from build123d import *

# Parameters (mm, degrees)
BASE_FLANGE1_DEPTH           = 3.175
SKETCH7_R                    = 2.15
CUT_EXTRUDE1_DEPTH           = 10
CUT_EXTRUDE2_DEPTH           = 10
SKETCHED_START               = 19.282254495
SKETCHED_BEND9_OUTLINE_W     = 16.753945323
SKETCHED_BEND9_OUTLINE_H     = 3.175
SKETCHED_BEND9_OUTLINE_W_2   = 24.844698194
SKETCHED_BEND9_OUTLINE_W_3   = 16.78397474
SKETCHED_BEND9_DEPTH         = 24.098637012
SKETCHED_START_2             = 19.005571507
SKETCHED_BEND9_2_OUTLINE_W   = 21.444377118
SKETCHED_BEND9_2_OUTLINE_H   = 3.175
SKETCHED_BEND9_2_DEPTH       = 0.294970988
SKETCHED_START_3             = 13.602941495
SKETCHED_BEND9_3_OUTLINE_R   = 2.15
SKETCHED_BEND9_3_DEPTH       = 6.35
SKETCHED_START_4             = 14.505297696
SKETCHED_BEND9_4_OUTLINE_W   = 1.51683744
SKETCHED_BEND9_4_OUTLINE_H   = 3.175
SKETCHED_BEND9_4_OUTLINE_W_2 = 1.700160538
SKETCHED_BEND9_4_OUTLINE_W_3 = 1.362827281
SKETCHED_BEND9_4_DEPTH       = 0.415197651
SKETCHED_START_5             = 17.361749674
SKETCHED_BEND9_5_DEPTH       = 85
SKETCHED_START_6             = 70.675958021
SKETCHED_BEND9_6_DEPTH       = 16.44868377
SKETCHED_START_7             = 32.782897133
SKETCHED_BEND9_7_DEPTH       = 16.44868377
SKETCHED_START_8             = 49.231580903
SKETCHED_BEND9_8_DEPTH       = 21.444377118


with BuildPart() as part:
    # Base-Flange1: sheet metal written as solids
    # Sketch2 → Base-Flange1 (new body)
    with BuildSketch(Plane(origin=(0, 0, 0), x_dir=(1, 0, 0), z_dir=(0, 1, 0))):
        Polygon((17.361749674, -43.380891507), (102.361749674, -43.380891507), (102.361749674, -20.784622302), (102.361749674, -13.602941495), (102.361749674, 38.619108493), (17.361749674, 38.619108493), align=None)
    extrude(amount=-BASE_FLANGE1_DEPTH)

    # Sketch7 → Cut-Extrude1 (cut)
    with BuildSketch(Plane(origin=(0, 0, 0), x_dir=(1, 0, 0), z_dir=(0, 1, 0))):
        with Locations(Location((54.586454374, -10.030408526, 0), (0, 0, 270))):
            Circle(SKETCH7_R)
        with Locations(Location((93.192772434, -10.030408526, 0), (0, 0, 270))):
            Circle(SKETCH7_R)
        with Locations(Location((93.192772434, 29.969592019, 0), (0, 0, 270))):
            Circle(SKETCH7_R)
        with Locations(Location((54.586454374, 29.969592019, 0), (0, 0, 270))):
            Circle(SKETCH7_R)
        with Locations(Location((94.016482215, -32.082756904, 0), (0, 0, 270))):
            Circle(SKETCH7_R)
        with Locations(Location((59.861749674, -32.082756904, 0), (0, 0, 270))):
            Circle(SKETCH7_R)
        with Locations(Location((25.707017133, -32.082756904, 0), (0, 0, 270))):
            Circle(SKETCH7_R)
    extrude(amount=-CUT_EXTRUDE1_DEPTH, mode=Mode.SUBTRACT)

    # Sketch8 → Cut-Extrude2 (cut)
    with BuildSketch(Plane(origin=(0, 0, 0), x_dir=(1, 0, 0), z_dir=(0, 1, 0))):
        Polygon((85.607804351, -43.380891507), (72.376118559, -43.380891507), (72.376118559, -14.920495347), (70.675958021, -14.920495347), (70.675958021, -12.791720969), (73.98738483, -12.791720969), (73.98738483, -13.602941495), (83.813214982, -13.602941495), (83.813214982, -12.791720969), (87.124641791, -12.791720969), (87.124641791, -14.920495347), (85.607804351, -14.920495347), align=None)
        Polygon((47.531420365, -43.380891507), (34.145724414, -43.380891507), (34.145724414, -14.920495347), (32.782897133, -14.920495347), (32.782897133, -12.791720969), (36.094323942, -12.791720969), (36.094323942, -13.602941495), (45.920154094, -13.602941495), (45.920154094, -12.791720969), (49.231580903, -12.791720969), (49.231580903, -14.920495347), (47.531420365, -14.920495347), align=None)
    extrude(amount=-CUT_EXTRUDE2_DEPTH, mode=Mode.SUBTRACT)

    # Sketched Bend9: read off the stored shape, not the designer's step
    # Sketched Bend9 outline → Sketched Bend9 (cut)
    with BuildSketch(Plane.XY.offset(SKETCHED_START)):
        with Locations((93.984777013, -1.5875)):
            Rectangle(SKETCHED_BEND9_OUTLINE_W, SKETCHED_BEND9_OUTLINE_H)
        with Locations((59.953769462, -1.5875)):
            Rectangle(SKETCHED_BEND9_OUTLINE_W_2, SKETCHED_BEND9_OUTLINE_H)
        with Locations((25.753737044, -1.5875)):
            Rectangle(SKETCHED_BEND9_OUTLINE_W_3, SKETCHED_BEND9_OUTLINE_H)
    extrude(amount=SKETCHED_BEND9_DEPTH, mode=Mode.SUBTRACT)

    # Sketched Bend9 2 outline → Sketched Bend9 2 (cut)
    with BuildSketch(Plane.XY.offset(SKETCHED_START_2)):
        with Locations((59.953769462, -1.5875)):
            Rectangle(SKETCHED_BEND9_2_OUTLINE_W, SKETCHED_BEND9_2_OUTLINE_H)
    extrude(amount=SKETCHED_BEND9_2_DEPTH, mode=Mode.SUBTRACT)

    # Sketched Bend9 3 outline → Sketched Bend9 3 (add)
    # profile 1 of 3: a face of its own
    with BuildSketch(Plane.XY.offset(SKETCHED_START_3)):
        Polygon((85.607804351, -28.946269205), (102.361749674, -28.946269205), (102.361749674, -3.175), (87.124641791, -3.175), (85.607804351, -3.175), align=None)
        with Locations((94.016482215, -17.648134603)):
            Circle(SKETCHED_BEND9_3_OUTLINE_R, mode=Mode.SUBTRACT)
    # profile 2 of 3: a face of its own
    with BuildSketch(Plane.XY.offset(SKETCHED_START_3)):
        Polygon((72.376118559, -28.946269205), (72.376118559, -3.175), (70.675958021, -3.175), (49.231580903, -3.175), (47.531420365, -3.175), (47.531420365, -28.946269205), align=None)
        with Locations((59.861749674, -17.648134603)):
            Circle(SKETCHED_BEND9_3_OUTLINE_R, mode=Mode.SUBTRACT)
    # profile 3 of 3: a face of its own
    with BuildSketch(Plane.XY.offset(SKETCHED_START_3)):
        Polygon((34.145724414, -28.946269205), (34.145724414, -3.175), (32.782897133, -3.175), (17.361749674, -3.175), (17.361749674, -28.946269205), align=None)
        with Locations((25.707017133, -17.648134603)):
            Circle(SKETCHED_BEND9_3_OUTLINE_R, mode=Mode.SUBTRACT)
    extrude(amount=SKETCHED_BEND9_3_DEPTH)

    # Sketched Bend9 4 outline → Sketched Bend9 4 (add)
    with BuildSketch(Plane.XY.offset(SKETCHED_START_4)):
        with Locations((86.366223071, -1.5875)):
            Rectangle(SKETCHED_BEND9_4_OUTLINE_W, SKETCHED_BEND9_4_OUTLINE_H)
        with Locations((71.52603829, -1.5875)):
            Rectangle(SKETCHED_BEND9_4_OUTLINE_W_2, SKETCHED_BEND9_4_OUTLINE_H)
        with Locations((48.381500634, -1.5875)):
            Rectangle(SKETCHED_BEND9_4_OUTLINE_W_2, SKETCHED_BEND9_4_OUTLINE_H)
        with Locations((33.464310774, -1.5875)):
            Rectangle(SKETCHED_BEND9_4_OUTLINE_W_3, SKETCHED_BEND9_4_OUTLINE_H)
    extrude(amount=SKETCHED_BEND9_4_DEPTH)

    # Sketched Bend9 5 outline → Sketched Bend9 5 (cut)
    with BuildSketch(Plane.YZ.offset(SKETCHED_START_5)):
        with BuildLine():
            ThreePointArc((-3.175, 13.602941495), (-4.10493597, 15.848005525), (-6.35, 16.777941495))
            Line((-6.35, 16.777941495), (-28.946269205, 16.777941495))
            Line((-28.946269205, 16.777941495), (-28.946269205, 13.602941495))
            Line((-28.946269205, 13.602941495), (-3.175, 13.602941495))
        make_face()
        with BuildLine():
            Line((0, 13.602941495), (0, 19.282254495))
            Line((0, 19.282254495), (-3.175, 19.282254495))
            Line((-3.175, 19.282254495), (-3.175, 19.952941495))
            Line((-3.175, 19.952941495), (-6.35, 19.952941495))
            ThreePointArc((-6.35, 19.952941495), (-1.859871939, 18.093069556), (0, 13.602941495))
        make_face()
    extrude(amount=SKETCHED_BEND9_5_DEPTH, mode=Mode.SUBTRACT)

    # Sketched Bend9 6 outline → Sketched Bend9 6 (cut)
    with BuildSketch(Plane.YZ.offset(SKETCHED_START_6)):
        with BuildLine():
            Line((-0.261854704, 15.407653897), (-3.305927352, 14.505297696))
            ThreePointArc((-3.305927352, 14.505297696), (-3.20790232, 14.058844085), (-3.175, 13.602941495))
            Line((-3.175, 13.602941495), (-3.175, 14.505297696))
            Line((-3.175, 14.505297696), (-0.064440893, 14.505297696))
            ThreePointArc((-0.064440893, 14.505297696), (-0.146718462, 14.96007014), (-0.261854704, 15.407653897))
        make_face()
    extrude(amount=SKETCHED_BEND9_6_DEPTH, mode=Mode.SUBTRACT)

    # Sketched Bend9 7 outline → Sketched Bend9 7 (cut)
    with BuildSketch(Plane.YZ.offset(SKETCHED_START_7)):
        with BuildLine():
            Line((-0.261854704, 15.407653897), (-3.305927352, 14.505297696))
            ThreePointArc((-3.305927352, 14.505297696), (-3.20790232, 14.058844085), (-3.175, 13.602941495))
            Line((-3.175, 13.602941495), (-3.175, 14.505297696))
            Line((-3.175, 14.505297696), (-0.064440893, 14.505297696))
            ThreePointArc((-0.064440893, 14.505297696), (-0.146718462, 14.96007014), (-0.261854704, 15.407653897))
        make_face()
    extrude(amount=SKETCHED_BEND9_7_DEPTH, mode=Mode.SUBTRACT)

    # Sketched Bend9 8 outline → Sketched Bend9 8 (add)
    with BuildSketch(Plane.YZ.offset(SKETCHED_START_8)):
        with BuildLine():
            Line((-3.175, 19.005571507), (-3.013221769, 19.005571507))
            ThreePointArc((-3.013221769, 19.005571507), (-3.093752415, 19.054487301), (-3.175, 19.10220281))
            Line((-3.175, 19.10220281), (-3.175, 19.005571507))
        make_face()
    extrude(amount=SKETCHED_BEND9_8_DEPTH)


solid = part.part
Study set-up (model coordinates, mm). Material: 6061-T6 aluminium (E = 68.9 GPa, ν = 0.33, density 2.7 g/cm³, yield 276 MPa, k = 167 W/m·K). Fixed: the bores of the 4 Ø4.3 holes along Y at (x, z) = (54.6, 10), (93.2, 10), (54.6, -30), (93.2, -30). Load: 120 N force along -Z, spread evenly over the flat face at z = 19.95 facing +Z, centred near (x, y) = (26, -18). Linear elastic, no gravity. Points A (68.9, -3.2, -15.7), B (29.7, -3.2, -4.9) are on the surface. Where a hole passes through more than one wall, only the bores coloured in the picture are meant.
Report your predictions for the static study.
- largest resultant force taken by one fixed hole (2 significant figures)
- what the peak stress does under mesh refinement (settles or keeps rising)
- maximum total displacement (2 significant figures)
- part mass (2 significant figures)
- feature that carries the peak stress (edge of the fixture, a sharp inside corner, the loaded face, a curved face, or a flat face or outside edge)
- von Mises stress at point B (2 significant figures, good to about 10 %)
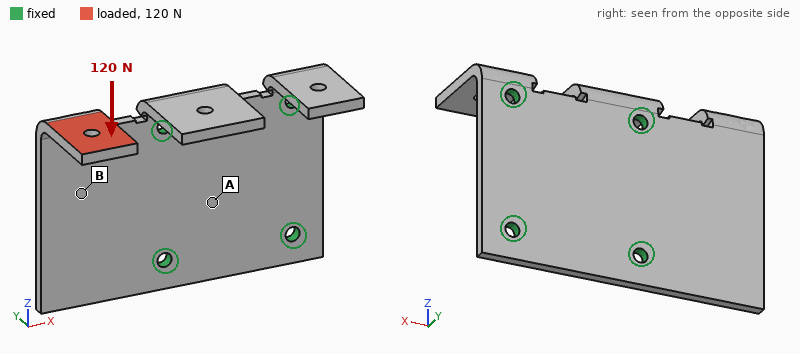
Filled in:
110 N
keeps rising
0.45 mm
52 g
a sharp inside corner
23 MPa
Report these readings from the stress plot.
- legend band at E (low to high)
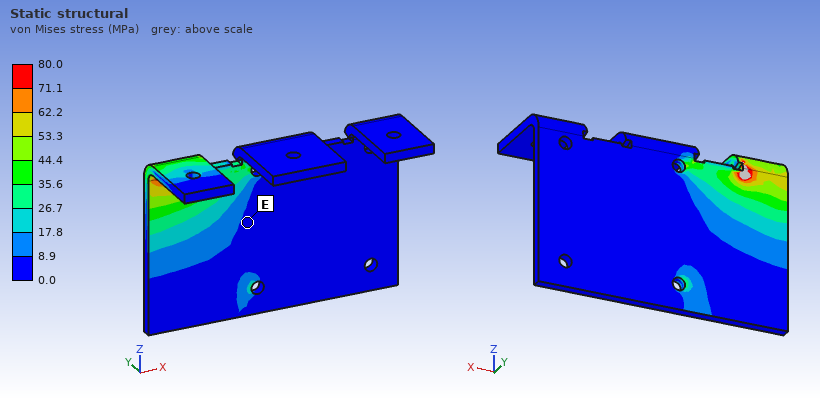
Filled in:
0.0 to 8.9 MPa
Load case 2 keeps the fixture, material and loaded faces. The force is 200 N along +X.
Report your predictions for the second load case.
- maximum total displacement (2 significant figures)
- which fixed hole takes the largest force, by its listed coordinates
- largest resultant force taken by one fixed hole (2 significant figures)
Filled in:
0.71 mm
(54.6, 10)
220 N
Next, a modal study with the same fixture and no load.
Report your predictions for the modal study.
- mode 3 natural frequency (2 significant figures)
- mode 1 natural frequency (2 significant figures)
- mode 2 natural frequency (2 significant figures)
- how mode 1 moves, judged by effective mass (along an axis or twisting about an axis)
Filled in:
2400 Hz
1200 Hz
1700 Hz
along Y
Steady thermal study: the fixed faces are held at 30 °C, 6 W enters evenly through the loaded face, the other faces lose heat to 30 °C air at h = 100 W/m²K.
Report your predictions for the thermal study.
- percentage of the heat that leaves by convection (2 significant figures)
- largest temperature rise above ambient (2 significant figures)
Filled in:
46 %
20 K
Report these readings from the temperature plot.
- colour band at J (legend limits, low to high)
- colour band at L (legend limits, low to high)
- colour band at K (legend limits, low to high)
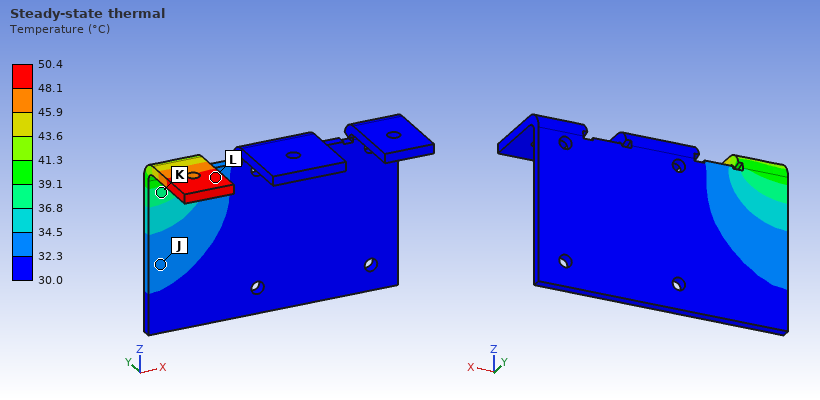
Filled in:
32.3 to 34.5 °C
48.1 to 50.4 °C
36.8 to 39.1 °C
